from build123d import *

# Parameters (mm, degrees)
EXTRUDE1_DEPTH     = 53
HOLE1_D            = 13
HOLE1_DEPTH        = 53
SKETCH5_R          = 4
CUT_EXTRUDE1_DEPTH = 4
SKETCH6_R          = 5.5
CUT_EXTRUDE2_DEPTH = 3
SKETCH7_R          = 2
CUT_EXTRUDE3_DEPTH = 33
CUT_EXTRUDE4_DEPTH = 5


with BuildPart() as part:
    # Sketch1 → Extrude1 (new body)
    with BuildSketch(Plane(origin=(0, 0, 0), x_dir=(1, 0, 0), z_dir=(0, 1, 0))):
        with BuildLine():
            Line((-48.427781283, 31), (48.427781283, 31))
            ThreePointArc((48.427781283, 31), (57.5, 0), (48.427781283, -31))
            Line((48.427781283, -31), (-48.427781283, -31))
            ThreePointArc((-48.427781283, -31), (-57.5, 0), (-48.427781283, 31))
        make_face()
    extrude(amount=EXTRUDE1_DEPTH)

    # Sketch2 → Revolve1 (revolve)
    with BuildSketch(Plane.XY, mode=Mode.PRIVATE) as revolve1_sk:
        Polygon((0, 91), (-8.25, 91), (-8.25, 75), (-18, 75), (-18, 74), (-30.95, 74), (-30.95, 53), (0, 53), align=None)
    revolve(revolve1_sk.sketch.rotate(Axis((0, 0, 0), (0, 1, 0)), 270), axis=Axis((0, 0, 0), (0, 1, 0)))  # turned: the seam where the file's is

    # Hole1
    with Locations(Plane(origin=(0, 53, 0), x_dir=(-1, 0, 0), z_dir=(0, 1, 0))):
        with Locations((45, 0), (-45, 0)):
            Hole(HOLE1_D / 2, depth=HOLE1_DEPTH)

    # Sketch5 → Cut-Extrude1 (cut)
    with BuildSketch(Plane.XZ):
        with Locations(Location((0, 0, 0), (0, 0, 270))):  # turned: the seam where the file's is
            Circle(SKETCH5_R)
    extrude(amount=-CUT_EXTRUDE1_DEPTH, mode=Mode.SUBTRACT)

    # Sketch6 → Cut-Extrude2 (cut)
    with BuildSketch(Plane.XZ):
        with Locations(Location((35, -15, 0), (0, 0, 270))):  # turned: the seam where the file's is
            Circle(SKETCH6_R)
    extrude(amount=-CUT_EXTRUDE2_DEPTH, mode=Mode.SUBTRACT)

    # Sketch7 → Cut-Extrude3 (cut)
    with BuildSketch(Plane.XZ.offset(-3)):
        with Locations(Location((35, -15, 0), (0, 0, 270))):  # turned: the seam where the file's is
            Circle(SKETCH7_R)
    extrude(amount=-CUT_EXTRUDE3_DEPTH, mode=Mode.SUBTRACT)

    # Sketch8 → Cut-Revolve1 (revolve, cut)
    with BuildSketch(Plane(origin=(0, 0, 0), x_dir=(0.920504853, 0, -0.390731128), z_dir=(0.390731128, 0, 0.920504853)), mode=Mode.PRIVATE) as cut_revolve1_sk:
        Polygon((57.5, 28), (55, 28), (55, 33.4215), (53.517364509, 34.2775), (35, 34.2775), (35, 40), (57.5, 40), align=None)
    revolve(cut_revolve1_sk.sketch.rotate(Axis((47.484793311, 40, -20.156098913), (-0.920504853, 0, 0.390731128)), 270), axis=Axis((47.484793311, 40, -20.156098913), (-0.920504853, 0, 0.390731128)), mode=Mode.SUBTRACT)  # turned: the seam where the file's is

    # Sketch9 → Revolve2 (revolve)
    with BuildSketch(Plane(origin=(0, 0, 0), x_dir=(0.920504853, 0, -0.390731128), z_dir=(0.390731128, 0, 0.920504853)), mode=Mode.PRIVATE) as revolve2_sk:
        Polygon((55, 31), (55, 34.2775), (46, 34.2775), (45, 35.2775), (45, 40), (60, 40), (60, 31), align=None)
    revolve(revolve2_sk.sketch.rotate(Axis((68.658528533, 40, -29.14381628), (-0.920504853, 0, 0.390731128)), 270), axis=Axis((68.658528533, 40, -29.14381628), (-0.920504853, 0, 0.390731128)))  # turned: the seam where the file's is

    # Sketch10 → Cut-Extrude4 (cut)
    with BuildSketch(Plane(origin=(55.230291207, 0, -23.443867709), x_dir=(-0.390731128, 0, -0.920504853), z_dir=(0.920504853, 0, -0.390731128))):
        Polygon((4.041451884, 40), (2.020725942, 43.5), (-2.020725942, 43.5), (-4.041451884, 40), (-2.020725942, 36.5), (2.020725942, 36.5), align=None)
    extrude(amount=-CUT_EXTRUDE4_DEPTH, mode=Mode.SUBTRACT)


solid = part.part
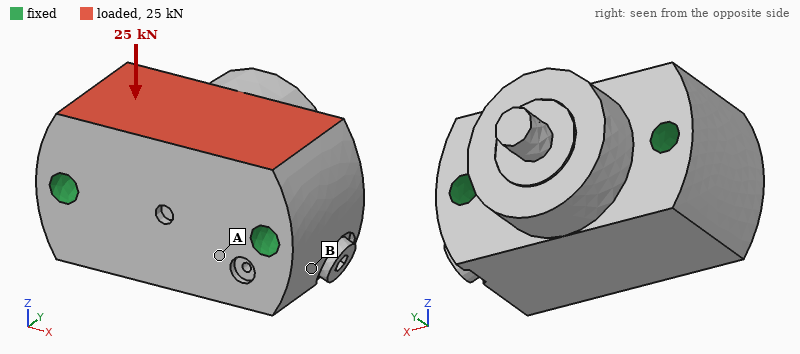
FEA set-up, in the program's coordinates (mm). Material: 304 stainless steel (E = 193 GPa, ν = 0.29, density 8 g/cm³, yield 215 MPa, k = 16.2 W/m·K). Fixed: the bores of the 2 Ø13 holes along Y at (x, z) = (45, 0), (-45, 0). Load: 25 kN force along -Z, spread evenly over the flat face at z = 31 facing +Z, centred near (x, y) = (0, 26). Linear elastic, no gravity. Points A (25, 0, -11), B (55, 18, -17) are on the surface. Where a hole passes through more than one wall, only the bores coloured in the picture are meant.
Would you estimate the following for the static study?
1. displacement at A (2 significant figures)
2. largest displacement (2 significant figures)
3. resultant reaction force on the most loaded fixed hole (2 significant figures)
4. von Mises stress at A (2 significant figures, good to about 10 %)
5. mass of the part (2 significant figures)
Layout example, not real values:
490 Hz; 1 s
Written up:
1.2 µm; 2.4 µm; 13 kN; 5.3 MPa; 3.3 kg
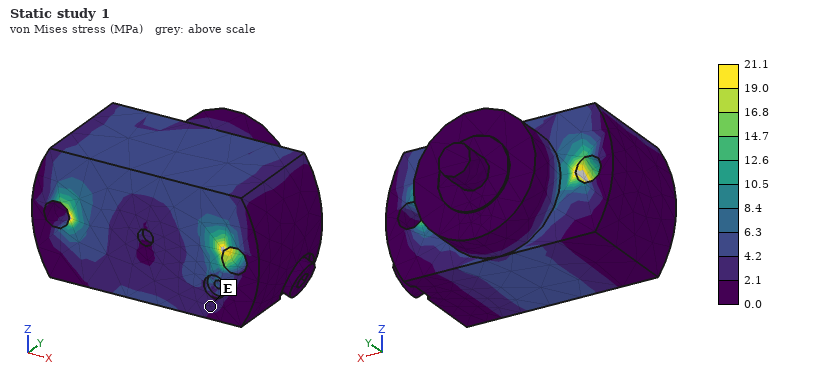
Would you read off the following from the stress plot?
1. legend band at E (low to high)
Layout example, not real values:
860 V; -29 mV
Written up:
2.1 to 4.2 MPa
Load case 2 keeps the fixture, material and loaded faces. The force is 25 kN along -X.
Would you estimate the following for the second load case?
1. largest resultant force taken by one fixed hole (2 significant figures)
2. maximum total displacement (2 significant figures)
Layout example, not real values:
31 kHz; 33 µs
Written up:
15 kN; 2.5 µm
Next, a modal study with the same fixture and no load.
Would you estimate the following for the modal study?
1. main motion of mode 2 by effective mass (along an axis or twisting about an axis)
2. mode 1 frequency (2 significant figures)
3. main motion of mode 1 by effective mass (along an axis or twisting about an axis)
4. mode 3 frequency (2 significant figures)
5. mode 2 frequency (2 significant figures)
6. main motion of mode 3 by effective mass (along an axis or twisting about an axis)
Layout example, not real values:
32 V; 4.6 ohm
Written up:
along Y; 8400 Hz; along Z; 13 kHz; 12 kHz; along Z
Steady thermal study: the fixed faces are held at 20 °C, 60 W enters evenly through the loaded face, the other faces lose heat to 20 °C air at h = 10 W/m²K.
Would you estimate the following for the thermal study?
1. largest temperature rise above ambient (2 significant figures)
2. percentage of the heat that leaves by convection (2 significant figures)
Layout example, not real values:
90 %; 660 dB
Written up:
29 K; 4.4 %
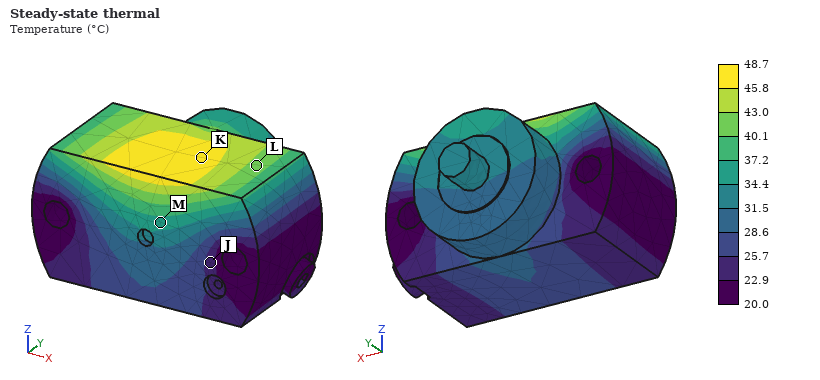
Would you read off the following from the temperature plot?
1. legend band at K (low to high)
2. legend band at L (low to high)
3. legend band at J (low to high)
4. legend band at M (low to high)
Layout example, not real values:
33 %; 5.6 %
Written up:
45.8 to 48.7 °C; 40.1 to 43.0 °C; 22.9 to 25.7 °C; 34.4 to 37.2 °C
